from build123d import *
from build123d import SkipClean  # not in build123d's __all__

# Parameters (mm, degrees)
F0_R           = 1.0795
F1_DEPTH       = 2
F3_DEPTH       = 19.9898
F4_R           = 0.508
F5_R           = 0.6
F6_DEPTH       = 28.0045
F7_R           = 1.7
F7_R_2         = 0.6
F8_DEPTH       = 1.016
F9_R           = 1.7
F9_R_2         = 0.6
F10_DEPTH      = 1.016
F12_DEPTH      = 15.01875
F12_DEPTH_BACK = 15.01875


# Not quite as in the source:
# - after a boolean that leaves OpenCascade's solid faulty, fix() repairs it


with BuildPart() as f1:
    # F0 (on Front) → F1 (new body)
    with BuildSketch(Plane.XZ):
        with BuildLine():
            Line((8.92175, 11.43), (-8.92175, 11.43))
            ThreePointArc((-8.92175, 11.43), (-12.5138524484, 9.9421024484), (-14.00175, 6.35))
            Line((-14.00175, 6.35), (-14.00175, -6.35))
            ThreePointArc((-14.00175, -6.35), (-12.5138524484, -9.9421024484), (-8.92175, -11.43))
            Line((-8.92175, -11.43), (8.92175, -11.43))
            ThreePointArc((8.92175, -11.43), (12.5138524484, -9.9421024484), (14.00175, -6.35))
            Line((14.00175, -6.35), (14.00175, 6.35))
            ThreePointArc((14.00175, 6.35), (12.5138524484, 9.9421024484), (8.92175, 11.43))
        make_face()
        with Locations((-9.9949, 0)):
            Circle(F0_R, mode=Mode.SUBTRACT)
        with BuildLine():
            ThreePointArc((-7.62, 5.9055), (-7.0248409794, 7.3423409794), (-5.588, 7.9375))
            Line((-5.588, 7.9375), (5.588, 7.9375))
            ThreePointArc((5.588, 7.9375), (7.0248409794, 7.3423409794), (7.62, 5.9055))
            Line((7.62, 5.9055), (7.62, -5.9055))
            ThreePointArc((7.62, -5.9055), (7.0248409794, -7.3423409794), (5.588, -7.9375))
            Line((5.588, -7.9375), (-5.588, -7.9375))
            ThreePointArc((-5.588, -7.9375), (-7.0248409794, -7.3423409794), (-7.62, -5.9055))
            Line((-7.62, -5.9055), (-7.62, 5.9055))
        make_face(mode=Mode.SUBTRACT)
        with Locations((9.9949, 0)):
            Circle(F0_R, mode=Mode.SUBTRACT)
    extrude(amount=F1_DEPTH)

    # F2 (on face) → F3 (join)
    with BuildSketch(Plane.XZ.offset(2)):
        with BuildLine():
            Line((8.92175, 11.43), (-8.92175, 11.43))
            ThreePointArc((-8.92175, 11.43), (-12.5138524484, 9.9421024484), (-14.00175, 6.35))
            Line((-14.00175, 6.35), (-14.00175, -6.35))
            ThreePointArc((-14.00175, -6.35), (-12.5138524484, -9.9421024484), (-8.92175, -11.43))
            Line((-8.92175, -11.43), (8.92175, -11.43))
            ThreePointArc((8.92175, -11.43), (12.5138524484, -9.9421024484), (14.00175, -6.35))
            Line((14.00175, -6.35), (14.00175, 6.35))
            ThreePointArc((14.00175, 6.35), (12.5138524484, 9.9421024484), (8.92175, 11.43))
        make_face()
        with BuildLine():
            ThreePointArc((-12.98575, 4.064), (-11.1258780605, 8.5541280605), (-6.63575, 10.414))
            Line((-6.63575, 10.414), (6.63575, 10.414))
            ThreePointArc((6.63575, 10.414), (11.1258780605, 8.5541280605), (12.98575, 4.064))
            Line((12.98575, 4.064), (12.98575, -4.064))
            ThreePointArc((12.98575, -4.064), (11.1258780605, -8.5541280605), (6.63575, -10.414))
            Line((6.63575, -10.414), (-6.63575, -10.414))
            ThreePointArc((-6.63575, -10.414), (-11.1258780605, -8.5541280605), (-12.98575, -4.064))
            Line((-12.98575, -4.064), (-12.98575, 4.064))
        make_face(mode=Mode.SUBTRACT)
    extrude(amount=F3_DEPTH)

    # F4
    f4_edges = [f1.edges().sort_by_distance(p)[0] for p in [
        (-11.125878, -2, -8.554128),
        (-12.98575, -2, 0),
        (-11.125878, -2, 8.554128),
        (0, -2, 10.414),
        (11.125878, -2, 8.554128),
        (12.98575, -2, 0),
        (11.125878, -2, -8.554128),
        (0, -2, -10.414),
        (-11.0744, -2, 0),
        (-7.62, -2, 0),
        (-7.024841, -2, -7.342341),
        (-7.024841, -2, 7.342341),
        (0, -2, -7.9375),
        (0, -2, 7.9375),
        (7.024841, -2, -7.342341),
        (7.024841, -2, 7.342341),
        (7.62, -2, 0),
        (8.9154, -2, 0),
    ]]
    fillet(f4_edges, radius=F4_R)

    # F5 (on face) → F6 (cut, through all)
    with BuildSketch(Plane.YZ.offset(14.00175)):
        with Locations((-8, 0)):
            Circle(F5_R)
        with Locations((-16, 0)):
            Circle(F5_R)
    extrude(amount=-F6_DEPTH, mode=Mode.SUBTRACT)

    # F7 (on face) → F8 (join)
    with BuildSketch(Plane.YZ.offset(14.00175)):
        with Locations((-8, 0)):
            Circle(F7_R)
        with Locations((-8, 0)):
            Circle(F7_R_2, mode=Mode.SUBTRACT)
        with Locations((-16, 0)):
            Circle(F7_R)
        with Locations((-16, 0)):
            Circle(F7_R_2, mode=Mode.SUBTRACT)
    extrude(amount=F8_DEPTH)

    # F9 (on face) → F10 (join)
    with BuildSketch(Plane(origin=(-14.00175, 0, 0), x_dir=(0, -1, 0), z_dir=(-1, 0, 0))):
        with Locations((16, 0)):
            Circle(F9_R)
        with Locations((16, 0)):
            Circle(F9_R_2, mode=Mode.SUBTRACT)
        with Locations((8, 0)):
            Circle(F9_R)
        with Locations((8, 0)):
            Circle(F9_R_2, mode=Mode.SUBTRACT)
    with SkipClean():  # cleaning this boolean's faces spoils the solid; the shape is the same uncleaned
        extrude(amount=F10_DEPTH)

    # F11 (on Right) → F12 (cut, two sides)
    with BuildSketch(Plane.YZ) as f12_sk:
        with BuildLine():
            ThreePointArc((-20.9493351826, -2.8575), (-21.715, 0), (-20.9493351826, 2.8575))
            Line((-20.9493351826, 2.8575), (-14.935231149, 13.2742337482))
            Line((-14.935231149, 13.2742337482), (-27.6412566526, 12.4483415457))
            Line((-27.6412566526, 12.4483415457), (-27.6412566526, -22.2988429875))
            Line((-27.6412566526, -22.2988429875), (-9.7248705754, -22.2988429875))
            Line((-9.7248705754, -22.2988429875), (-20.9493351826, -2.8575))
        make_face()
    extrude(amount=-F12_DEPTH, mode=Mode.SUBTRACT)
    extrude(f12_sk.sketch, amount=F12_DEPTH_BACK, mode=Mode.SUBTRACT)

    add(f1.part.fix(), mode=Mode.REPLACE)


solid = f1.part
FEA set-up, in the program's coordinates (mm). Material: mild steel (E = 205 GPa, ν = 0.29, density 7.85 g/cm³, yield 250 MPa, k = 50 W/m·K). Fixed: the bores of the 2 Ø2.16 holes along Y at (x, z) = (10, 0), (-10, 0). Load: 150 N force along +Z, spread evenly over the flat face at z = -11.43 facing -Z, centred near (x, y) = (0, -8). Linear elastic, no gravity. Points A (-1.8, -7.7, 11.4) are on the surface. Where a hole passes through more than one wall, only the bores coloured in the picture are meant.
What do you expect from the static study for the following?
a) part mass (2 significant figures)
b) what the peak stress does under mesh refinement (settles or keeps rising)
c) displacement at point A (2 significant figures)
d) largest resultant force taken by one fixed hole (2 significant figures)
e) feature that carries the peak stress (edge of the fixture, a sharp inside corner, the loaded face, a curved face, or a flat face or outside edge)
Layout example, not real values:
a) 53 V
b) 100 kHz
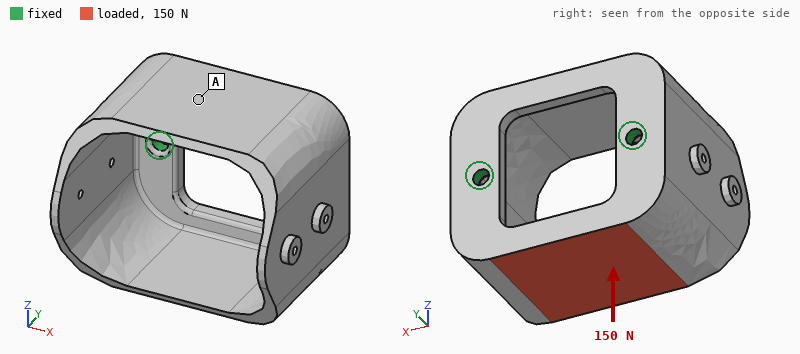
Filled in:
a) 20 g
b) keeps rising
c) 9.2 µm
d) 88 N
e) edge of the fixture
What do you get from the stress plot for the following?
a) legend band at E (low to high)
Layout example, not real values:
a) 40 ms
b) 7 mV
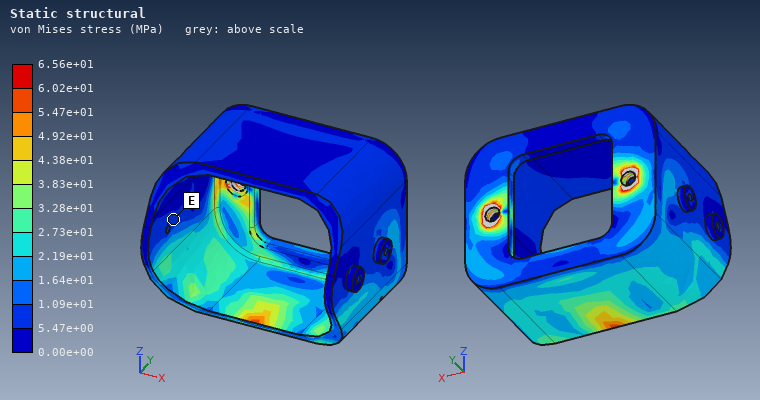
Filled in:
a) 5.47e+00 to 1.09e+01 MPa
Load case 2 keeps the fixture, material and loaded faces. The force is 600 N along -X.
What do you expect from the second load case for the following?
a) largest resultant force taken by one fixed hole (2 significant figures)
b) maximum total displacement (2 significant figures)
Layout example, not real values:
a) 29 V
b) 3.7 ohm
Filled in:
a) 390 N
b) 37 µm
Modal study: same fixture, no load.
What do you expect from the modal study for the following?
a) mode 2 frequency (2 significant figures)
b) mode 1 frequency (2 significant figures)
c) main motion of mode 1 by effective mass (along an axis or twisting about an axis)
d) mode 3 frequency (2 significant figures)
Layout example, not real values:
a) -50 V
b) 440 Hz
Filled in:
a) 5300 Hz
b) 3500 Hz
c) along Z
d) 8000 Hz
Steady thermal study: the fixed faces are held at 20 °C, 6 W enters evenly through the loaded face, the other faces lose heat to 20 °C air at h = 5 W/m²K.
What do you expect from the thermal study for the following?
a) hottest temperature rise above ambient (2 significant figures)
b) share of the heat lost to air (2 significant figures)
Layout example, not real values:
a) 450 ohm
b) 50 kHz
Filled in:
a) 45 K
b) 5.1 %
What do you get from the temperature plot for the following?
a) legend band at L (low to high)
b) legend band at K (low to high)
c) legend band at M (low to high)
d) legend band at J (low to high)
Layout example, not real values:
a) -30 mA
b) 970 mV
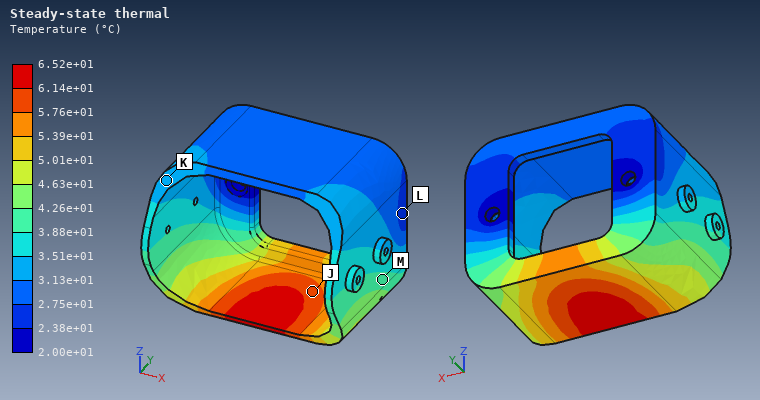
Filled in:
a) 2.38e+01 to 2.75e+01 °C
b) 3.13e+01 to 3.51e+01 °C
c) 3.88e+01 to 4.26e+01 °C
d) 5.76e+01 to 6.14e+01 °C
